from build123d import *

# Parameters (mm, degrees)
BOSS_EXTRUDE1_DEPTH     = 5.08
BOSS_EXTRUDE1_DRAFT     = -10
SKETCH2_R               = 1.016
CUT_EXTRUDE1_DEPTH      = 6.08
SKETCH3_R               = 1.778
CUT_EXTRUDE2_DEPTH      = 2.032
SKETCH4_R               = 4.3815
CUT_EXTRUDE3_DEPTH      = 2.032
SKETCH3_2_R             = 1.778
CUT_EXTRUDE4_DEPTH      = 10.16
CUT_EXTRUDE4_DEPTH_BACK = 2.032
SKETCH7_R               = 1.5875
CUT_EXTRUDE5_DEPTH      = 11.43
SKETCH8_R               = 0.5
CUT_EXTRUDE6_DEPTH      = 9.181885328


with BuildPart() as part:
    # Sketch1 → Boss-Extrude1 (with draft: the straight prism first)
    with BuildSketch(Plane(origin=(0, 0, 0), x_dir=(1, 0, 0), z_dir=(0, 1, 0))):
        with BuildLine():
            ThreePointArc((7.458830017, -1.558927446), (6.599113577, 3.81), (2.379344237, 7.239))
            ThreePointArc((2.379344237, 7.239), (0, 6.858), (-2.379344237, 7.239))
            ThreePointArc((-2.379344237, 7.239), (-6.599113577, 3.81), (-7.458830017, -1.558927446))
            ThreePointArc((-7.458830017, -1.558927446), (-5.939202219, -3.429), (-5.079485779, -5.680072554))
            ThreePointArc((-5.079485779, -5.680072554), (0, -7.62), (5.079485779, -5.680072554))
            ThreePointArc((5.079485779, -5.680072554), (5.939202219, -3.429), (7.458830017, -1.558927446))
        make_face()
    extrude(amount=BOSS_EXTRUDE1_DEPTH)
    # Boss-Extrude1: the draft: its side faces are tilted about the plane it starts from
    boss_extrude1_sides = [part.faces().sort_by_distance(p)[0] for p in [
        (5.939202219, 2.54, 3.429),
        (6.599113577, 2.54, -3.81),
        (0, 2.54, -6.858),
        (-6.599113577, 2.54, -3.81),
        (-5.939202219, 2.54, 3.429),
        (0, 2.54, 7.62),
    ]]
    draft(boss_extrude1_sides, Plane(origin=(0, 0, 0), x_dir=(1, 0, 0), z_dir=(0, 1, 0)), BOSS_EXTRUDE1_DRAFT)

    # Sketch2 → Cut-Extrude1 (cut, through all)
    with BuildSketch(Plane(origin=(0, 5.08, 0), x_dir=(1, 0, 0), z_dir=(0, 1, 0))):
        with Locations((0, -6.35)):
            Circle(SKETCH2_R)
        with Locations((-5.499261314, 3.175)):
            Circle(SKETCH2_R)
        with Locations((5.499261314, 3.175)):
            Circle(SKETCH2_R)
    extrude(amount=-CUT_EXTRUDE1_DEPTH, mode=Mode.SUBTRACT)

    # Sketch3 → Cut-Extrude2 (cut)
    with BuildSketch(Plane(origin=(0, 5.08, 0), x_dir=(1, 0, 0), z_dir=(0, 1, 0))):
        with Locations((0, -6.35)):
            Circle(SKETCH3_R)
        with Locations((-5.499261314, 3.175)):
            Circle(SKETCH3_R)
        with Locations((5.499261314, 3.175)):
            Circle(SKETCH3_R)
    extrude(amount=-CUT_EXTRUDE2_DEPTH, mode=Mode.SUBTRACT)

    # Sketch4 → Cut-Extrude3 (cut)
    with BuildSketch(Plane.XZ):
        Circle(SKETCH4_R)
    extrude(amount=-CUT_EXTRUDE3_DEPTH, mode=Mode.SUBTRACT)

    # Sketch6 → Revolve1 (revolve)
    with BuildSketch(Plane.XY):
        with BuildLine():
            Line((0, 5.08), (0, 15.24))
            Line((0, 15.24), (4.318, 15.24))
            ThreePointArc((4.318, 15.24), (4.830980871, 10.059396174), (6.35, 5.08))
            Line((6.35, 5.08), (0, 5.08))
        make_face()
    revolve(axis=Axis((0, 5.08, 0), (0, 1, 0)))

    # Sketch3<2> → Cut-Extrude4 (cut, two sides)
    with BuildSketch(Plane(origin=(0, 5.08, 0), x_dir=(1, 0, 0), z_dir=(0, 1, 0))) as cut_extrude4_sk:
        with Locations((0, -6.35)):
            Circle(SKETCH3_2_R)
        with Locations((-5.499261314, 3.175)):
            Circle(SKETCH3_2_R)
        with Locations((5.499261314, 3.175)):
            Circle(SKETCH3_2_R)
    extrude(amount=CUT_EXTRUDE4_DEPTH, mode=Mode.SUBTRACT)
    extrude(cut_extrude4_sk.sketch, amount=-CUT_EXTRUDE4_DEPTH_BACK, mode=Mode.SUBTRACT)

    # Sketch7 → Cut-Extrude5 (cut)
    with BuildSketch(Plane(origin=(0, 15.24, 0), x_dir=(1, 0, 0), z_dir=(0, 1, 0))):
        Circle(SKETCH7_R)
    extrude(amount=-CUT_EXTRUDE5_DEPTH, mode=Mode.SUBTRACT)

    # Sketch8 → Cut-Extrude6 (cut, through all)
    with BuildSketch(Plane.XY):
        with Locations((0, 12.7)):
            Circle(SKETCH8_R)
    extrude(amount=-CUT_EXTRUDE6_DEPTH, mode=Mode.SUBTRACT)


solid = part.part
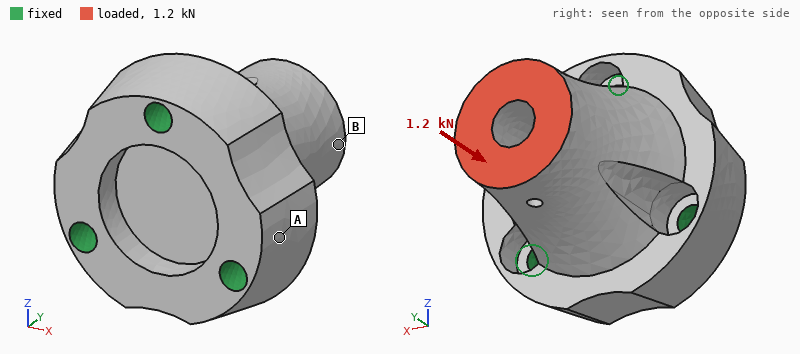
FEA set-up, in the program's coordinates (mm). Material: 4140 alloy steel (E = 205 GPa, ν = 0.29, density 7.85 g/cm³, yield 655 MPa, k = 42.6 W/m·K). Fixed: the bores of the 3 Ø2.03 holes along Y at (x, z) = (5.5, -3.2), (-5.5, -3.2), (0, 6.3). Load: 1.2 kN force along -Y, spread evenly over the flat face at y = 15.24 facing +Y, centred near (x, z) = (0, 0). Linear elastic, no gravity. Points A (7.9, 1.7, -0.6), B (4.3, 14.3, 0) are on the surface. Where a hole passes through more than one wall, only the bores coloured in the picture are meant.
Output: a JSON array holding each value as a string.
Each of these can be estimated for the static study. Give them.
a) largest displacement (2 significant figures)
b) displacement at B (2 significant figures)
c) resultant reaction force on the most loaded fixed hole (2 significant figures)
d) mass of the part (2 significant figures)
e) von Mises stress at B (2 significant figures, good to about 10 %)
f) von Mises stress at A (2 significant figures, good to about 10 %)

["1.8 µm", "1.6 µm", "420 N", "12 g", "23 MPa", "9.7 MPa"]
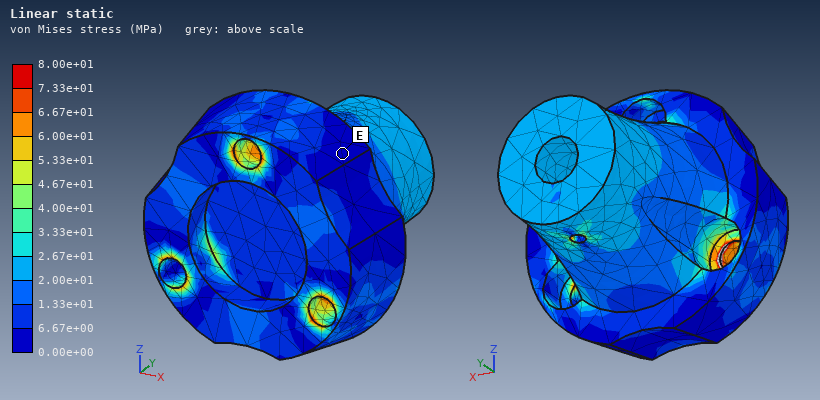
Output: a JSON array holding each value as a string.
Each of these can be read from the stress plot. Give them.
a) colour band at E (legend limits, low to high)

["0.00e+00 to 6.67e+00 MPa"]
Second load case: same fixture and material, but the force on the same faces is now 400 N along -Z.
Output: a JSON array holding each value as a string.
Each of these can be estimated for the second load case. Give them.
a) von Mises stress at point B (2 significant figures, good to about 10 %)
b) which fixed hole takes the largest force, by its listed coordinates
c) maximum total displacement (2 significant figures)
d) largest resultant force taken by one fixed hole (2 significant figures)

["13 MPa", "(0, 6.3)", "5.1 µm", "550 N"]
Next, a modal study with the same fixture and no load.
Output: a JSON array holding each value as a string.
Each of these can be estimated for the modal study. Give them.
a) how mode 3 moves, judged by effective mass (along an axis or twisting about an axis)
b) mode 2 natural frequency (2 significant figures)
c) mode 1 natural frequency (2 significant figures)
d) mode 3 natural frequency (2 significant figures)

["along Y", "33 kHz", "33 kHz", "61 kHz"]
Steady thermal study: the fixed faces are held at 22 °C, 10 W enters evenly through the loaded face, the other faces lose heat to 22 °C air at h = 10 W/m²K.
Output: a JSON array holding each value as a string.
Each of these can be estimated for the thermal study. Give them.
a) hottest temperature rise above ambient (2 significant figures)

["51 K"]
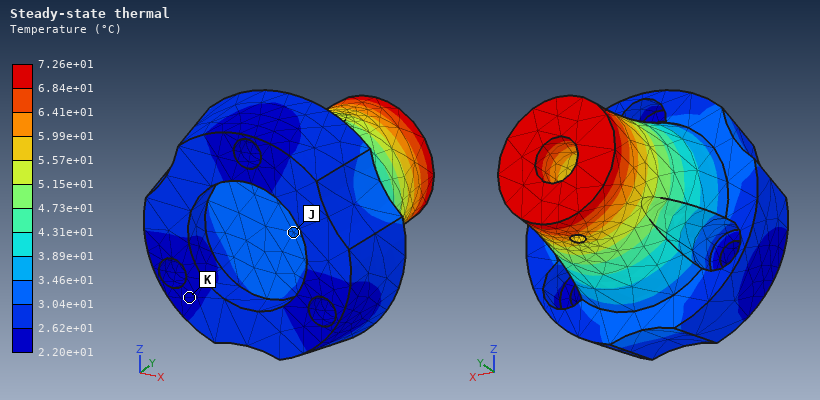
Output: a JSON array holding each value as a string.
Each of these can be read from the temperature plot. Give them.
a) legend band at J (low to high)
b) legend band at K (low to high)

["3.04e+01 to 3.46e+01 °C", "2.20e+01 to 2.62e+01 °C"]
